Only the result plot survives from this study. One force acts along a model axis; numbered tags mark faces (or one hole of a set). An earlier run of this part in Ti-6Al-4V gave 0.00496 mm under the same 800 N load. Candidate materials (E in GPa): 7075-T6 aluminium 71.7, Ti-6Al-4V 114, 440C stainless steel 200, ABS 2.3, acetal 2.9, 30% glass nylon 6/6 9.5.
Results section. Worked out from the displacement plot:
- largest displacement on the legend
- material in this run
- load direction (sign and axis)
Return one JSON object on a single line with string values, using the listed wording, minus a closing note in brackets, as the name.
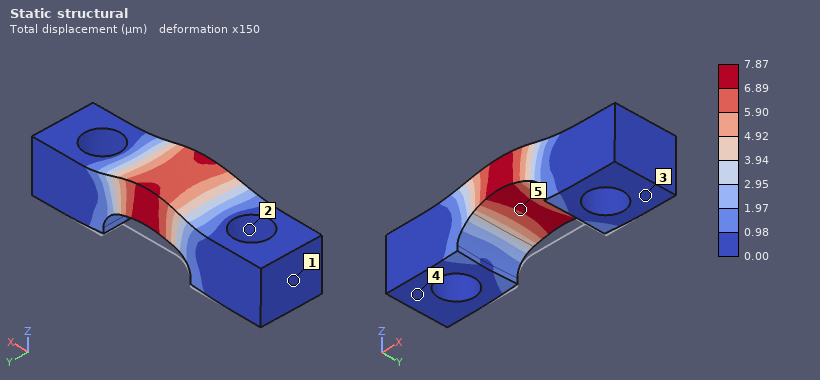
{"largest displacement on the legend": "7.87 µm", "material in this run": "7075-T6 aluminium", "load direction": "+Z"}
